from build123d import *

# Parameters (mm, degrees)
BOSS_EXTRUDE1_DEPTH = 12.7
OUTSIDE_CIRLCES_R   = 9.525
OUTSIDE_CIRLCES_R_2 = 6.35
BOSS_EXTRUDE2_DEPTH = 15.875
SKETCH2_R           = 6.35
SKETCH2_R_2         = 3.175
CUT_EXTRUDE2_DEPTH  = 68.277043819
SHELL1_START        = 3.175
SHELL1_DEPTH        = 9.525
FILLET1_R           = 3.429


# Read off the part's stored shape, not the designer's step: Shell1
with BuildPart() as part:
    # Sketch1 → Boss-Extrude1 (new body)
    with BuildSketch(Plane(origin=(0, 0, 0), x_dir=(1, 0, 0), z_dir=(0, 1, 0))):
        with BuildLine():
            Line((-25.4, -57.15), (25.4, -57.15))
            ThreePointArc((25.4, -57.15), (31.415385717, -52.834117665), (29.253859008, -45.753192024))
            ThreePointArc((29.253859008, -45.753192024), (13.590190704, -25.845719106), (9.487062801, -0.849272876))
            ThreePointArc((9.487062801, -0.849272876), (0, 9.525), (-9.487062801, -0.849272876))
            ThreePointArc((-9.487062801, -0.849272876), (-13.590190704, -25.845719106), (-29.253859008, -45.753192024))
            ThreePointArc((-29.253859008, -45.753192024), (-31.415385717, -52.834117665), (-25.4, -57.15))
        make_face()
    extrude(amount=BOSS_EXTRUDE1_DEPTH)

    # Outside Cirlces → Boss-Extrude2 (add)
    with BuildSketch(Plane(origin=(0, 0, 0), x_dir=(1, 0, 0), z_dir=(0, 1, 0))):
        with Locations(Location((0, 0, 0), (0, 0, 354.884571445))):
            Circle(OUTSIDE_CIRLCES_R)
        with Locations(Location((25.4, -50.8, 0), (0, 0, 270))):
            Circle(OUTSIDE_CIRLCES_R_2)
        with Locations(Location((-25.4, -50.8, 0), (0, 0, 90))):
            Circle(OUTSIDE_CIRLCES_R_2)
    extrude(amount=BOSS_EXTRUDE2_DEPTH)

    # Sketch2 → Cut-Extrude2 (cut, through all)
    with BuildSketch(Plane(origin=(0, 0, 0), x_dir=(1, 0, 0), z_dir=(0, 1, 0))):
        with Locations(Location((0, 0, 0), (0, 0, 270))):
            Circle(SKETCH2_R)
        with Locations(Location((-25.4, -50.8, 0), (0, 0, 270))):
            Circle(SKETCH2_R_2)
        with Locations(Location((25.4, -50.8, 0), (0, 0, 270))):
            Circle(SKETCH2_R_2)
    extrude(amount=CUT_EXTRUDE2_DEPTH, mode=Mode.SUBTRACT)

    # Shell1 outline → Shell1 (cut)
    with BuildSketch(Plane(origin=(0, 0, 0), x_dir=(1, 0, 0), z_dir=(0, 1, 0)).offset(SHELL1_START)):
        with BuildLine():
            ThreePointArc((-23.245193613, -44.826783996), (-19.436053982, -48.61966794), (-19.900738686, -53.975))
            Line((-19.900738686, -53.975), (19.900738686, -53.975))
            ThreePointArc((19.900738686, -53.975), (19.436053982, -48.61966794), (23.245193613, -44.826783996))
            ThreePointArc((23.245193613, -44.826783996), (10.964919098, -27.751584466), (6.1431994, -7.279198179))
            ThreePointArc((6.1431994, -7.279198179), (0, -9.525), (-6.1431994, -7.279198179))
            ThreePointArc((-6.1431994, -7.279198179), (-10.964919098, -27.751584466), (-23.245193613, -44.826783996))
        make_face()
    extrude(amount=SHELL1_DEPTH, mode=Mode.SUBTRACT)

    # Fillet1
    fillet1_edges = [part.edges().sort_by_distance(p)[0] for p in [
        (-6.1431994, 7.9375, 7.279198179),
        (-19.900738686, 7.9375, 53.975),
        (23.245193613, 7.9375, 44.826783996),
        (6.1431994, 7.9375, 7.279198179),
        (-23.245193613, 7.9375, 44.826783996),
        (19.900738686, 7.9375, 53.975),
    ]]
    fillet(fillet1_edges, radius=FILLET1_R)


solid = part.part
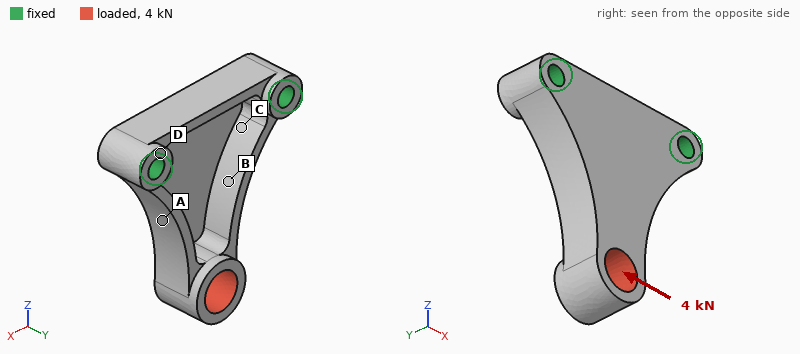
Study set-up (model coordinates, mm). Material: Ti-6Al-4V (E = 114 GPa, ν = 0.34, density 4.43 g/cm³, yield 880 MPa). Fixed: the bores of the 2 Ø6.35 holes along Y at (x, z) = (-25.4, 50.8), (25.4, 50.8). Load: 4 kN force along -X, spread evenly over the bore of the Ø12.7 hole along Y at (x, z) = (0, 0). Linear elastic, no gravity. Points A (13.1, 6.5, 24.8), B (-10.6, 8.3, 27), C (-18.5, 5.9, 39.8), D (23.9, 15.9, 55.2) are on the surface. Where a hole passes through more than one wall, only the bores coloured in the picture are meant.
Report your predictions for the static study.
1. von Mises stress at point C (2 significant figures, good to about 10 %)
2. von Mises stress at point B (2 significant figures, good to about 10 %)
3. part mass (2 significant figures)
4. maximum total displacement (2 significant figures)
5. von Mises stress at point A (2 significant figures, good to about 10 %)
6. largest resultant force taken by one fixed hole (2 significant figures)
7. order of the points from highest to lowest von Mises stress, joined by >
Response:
80 MPa
42 MPa
66 g
0.21 mm
170 MPa
4.5 kN
A > C > B > D
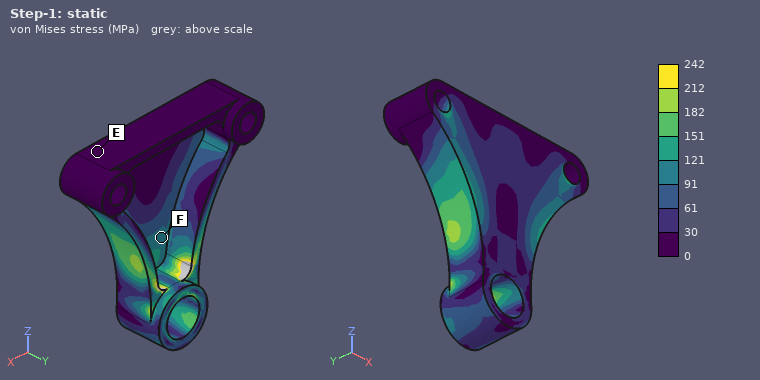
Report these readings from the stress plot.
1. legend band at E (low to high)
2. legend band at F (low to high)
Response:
0 to 30 MPa
91 to 121 MPa
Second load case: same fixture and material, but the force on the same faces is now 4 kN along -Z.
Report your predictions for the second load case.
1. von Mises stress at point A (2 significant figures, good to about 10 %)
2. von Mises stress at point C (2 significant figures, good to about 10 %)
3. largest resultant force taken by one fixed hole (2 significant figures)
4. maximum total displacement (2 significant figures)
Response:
75 MPa
71 MPa
2.3 kN
0.17 mm
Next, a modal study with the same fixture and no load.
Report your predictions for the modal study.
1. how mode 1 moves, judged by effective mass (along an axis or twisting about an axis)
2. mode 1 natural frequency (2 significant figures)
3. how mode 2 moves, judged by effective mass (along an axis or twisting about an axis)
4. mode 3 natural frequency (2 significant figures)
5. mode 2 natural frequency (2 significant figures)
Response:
along Y
2500 Hz
along X
8800 Hz
6400 Hz
